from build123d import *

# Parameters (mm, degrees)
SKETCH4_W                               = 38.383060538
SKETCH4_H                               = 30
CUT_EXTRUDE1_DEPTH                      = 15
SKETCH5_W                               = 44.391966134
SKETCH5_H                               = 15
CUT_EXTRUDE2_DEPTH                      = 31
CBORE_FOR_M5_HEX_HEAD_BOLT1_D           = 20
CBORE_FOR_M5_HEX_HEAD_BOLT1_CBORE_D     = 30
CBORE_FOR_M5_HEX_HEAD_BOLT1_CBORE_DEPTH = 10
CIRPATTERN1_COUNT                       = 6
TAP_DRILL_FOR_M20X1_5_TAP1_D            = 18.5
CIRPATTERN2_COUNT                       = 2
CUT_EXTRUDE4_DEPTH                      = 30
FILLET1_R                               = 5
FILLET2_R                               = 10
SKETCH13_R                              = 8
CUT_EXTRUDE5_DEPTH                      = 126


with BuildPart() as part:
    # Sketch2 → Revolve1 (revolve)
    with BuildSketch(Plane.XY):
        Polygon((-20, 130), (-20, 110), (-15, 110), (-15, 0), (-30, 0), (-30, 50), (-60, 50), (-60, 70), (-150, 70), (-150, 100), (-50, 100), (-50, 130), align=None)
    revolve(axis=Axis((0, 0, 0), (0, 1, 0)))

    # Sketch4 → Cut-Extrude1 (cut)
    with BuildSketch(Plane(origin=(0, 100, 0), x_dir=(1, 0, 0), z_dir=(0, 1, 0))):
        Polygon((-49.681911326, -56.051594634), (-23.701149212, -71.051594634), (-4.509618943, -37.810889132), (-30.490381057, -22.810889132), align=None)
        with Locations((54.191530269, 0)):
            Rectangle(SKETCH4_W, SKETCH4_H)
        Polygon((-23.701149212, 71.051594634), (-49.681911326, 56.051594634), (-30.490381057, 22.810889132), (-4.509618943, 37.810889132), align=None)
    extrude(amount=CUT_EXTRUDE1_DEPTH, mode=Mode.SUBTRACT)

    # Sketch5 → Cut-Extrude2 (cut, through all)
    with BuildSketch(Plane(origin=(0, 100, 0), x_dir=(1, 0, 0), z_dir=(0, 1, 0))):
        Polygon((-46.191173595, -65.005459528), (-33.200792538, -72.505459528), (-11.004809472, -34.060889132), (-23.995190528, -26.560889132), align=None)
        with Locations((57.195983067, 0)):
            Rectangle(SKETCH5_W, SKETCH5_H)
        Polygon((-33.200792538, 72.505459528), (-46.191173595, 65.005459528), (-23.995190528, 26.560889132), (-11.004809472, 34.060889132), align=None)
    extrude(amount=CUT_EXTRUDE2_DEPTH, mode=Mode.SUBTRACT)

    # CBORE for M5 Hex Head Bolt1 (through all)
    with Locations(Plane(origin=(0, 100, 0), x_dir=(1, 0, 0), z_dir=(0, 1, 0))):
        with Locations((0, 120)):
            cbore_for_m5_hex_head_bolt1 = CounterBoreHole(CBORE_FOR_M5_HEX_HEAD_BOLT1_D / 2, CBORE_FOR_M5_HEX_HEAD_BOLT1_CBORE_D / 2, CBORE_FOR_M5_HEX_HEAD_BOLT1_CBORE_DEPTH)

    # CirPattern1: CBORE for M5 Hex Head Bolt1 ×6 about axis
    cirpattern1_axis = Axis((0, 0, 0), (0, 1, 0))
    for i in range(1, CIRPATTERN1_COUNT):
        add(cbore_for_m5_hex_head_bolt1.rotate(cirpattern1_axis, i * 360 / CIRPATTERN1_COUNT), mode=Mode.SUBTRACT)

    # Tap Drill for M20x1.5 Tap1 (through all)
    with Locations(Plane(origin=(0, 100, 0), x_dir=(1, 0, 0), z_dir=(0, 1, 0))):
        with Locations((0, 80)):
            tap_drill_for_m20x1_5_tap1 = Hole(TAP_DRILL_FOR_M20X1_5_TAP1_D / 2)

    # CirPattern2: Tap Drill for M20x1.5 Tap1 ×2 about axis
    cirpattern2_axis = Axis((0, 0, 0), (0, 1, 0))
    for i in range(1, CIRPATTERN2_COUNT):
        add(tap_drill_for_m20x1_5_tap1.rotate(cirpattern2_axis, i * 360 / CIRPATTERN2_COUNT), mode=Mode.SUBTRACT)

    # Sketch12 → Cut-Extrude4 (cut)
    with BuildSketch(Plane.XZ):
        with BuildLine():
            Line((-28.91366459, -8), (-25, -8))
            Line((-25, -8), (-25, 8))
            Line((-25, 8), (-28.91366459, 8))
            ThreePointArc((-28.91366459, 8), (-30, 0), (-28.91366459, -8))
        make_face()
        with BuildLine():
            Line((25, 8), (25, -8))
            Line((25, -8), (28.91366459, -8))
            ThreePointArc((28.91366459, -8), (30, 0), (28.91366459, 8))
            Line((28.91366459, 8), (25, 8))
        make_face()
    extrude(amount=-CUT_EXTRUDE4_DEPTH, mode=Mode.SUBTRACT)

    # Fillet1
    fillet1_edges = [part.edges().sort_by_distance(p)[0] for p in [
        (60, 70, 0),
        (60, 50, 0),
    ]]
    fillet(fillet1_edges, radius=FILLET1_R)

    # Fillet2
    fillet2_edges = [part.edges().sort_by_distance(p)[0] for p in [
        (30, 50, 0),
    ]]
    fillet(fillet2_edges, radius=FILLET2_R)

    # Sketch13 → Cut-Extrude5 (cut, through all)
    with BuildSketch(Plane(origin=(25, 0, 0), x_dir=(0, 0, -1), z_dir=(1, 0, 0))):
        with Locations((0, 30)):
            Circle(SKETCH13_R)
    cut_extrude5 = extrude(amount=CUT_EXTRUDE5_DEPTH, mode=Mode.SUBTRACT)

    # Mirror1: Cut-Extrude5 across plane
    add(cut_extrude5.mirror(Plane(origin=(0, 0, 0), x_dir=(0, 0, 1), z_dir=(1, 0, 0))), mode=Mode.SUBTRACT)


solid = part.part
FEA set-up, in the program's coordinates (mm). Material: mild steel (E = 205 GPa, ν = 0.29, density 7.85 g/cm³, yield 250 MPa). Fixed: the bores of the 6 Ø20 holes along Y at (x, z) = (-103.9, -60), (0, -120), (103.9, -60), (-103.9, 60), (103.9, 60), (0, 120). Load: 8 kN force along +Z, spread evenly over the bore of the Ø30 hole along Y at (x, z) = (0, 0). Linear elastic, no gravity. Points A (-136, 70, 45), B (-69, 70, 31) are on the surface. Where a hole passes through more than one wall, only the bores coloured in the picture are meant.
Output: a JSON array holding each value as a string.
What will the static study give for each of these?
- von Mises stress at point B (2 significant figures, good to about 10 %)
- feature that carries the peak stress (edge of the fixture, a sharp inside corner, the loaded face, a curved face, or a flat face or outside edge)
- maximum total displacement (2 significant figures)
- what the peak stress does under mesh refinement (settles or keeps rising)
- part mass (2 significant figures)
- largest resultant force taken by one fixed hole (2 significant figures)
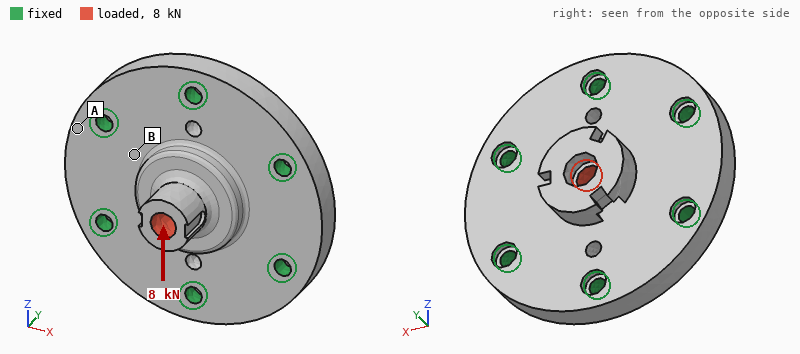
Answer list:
["1.6 MPa", "edge of the fixture", "3.5 µm", "keeps rising", "20 kg", "1.8 kN"]
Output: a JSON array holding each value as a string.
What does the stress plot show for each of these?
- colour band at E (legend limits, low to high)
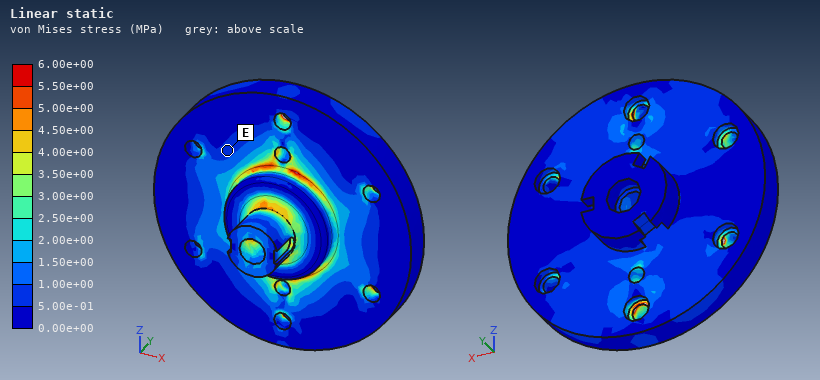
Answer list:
["5.00e-01 to 1.00e+00 MPa"]
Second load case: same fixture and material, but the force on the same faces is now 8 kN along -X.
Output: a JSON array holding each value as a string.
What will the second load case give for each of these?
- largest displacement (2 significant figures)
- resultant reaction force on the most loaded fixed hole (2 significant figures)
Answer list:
["3.5 µm", "1.8 kN"]
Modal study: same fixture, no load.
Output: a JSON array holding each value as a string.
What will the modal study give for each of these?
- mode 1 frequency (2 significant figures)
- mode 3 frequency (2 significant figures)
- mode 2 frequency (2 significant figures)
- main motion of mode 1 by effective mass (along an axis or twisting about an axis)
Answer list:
["3200 Hz", "5100 Hz", "5000 Hz", "along Y"]
